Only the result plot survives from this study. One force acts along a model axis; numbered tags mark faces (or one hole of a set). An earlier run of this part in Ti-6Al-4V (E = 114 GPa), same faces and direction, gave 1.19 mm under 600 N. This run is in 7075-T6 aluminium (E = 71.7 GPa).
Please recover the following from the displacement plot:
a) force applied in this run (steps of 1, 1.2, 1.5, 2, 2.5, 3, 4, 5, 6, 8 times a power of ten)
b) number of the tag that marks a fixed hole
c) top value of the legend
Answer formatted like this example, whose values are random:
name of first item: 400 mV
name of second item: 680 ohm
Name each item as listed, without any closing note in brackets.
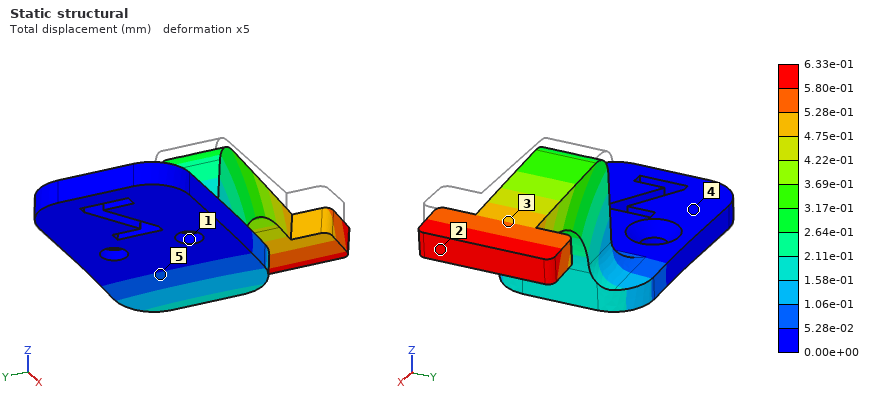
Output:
force applied in this run: 200 N
number of the tag that marks a fixed hole: 1
top value of the legend: 6.33e-01 mm
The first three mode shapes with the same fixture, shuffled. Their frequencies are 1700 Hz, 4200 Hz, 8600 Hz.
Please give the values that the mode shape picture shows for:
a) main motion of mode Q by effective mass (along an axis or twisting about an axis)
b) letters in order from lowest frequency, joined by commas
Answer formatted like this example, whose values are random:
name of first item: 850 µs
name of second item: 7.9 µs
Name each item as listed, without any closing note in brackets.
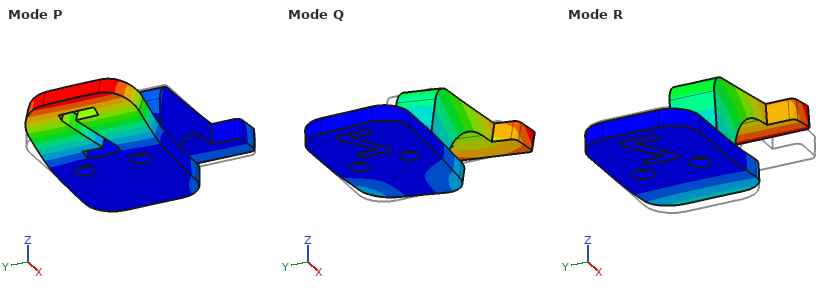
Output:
main motion of mode Q by effective mass: along Y
letters in order from lowest frequency, joined by commas: R, Q, P
